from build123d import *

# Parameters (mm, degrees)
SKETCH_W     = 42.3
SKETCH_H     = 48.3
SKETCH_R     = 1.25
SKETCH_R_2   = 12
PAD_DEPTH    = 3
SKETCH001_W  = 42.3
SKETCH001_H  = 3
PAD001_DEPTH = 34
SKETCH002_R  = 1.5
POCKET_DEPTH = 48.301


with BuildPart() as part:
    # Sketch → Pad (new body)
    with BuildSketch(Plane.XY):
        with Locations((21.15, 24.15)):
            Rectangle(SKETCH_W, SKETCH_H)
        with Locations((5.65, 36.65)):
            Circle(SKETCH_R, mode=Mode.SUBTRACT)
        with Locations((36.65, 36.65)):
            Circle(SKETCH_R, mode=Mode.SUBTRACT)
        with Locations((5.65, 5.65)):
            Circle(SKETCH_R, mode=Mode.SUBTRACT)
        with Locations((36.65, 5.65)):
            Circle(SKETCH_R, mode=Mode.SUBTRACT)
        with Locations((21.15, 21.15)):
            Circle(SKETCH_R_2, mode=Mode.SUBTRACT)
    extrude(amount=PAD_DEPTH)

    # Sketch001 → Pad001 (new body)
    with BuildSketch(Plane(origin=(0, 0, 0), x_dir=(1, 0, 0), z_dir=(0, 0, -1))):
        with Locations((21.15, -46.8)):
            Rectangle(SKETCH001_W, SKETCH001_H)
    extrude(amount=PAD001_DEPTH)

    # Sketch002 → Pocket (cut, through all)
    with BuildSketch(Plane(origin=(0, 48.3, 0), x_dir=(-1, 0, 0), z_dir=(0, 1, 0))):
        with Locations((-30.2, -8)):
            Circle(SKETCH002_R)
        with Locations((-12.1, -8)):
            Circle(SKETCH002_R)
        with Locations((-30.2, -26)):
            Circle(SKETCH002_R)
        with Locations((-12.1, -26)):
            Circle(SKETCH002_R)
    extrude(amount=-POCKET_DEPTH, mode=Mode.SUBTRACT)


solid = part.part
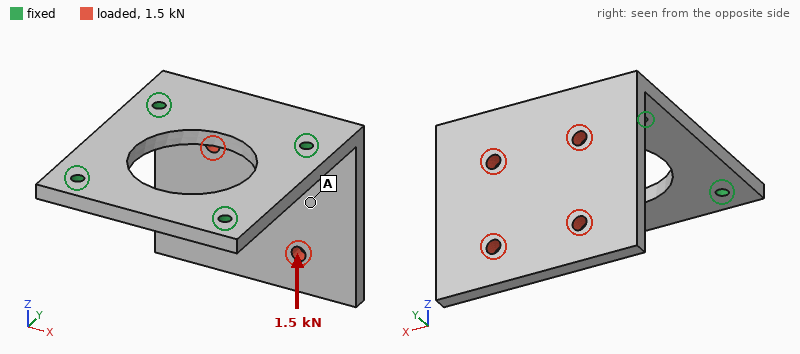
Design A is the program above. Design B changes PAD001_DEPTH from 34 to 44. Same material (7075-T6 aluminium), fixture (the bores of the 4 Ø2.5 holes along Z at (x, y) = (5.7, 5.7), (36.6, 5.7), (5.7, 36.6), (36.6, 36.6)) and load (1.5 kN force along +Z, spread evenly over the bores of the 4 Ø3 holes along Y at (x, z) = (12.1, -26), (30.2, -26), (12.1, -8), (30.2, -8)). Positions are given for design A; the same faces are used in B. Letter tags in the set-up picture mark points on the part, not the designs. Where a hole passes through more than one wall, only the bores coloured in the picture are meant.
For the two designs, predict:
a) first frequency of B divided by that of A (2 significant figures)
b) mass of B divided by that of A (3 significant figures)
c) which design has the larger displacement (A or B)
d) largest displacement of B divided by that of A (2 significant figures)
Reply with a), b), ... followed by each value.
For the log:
a) 0.65
b) 1.14
c) B
d) 1.3
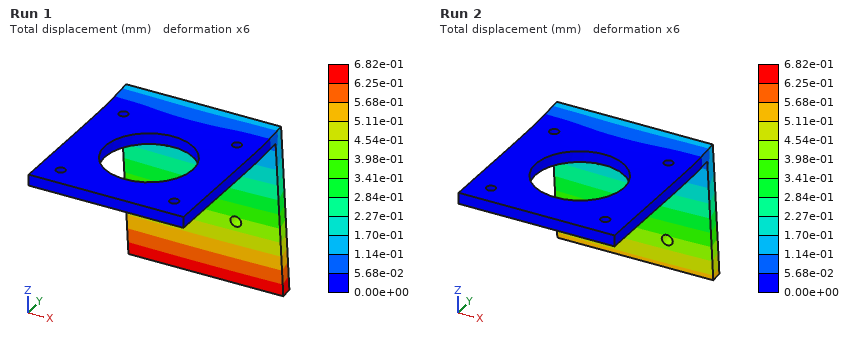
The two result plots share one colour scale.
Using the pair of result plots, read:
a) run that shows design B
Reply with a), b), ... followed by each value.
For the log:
a) Run 1
